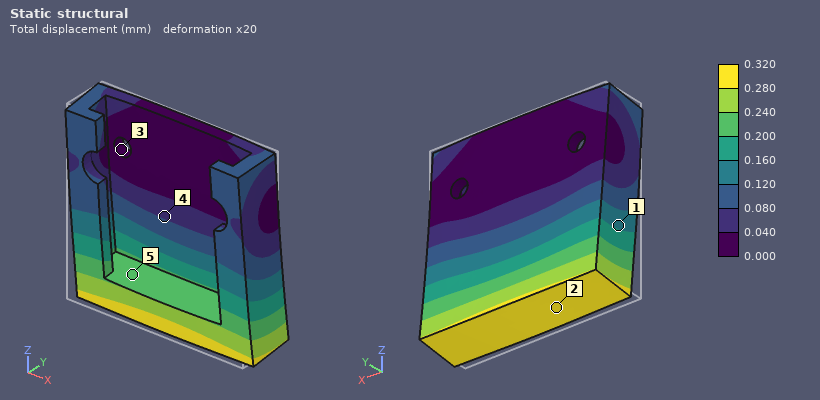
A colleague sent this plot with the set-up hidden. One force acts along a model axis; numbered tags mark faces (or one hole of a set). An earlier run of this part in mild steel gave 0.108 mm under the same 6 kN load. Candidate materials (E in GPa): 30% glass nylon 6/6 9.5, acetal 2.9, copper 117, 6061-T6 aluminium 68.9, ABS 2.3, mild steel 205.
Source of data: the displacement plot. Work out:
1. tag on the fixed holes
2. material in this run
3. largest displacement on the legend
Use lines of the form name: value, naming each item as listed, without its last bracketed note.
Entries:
tag on the fixed holes: 3
material in this run: 6061-T6 aluminium
largest displacement on the legend: 0.320 mm
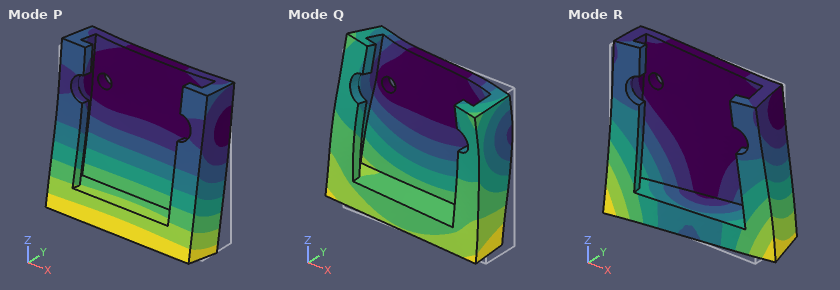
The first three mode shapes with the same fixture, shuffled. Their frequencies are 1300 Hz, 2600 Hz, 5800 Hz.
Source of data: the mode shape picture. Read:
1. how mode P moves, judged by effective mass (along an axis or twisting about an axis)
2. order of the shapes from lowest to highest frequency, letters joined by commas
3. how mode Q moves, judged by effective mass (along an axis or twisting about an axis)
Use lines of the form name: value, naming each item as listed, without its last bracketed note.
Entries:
how mode P moves, judged by effective mass: along Y
order of the shapes from lowest to highest frequency, letters joined by commas: P, R, Q
how mode Q moves, judged by effective mass: along X
